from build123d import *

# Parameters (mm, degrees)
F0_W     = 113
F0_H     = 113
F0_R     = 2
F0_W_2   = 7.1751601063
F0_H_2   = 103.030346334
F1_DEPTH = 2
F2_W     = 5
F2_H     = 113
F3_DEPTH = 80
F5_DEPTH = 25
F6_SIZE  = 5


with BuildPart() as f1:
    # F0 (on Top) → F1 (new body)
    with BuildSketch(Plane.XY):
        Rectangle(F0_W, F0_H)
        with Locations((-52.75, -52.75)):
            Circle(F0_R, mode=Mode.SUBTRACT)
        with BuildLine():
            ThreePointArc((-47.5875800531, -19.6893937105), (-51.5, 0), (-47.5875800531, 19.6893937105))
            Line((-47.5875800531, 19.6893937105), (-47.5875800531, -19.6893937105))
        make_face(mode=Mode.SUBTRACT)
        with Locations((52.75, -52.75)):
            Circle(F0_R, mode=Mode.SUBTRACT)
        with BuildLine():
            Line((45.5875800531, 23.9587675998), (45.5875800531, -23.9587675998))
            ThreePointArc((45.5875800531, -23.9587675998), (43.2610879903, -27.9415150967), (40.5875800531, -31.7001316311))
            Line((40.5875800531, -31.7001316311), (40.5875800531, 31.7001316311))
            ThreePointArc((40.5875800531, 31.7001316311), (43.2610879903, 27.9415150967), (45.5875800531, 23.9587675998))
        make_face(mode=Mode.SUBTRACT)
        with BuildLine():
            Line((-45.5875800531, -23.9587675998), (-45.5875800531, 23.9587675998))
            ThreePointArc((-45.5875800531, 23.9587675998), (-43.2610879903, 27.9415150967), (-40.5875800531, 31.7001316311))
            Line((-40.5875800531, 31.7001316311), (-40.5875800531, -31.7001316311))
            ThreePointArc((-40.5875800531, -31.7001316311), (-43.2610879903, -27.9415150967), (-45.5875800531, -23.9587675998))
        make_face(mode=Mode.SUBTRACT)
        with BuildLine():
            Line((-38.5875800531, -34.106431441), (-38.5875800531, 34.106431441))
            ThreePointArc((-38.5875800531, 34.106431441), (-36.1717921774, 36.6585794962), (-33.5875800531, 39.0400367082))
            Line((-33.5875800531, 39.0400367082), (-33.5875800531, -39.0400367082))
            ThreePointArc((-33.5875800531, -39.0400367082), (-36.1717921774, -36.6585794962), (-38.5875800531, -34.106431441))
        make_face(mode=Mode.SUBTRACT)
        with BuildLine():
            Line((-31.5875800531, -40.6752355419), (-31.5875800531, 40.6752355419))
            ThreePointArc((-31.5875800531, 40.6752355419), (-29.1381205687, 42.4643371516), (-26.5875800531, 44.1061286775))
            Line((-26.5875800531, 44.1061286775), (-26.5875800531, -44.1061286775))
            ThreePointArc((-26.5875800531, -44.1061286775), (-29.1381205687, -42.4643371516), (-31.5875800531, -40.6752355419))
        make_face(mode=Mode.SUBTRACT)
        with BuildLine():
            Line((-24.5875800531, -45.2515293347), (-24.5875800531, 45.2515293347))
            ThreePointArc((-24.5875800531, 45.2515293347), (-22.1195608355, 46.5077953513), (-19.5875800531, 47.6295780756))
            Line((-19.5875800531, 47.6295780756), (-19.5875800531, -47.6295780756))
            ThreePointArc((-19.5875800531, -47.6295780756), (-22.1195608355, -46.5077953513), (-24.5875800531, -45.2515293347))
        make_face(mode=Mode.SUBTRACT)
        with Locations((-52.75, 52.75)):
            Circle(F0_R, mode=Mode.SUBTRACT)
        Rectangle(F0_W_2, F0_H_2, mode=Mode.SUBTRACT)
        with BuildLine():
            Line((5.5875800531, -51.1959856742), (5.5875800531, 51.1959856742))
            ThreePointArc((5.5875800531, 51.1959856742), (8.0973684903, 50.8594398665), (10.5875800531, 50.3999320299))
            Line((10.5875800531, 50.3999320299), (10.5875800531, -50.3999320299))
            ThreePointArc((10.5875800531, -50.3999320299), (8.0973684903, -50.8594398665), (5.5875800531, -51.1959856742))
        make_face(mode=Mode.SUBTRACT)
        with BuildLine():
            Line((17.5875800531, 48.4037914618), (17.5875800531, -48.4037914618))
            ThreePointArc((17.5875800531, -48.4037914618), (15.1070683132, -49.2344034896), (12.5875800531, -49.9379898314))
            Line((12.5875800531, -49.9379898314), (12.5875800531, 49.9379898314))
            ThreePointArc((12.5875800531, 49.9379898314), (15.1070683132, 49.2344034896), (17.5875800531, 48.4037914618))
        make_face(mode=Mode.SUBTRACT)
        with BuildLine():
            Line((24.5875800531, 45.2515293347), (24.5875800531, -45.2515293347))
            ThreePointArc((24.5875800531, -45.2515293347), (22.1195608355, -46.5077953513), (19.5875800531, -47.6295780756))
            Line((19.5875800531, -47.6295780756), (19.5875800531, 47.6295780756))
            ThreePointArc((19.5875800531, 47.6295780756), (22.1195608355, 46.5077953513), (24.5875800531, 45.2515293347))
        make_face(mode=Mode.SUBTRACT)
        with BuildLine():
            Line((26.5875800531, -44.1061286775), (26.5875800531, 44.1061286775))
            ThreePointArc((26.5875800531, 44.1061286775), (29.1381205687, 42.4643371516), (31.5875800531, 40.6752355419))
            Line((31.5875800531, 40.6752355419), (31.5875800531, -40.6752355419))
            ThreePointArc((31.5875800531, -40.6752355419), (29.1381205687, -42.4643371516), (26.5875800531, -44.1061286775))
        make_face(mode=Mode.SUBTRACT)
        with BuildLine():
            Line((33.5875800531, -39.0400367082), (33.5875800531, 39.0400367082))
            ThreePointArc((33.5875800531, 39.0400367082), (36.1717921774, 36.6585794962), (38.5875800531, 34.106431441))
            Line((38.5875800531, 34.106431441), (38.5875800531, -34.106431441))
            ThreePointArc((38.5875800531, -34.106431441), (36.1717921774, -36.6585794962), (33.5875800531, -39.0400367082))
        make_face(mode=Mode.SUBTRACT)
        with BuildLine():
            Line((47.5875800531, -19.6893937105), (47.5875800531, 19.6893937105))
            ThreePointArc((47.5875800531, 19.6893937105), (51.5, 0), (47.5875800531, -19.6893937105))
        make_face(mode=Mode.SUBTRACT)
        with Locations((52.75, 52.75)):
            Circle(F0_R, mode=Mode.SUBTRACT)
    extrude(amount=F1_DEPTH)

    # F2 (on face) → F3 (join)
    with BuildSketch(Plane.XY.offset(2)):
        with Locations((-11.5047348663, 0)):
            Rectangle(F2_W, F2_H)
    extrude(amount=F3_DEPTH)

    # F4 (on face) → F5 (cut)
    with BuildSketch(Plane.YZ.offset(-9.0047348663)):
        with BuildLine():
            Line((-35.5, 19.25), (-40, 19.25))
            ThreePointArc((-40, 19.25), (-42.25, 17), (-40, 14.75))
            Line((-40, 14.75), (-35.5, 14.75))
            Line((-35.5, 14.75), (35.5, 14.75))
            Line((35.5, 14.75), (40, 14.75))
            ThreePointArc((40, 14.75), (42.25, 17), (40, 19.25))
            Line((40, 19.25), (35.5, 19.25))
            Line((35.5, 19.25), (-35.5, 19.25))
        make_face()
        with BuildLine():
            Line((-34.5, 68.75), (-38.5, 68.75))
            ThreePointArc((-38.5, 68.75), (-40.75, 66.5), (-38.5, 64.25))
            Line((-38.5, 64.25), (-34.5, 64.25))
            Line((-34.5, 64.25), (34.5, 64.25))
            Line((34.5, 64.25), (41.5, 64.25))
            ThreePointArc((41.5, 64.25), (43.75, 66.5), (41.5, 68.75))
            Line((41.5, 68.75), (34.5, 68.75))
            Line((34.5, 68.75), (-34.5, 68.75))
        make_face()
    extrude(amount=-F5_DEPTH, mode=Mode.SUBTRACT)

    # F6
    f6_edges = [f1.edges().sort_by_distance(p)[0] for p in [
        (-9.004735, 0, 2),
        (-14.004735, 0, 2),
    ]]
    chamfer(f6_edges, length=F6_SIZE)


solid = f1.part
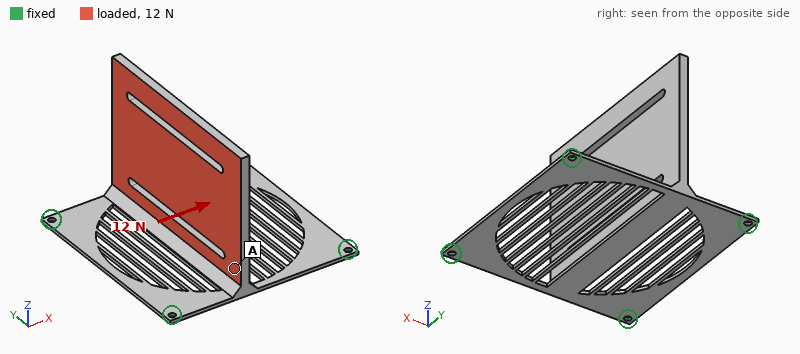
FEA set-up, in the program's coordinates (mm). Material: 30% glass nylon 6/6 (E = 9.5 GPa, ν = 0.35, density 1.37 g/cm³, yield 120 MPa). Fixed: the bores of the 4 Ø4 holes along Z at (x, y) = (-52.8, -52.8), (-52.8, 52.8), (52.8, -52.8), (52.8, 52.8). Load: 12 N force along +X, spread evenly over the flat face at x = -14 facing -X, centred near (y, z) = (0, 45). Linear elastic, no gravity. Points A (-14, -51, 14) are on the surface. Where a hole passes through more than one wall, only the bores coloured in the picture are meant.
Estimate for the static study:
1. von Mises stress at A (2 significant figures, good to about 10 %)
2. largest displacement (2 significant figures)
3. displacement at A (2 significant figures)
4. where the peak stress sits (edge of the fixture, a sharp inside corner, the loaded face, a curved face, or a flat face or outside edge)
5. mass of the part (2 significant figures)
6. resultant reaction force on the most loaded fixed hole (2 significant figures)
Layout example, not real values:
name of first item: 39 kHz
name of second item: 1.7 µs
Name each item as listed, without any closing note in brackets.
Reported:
von Mises stress at A: 2.7 MPa
largest displacement: 2.0 mm
displacement at A: 0.40 mm
where the peak stress sits: a flat face or outside edge
mass of the part: 82 g
resultant reaction force on the most loaded fixed hole: 5.4 N
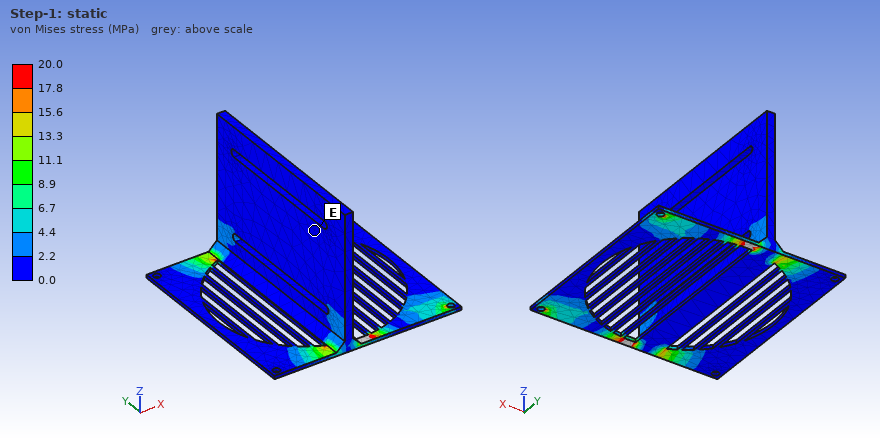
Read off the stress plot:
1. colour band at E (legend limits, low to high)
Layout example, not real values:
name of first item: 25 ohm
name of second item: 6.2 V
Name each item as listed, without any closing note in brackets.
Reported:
colour band at E: 0.0 to 2.2 MPa
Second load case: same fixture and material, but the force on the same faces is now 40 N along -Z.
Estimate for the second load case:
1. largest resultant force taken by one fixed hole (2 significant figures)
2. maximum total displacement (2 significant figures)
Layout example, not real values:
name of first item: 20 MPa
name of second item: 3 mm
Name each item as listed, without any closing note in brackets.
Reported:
largest resultant force taken by one fixed hole: 15 N
maximum total displacement: 1.9 mm
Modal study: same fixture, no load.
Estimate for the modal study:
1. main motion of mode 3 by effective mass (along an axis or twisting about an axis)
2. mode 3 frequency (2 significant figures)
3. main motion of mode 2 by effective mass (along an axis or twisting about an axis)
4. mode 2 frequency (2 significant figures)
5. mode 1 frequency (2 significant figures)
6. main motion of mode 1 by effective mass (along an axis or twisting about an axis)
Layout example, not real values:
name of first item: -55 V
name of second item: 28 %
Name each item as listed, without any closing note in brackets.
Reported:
main motion of mode 3 by effective mass: along Z
mode 3 frequency: 150 Hz
main motion of mode 2 by effective mass: along Y
mode 2 frequency: 140 Hz
mode 1 frequency: 62 Hz
main motion of mode 1 by effective mass: along X
